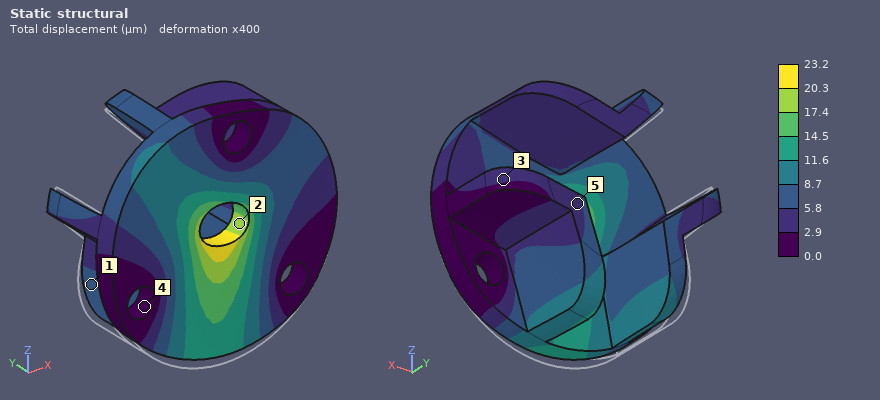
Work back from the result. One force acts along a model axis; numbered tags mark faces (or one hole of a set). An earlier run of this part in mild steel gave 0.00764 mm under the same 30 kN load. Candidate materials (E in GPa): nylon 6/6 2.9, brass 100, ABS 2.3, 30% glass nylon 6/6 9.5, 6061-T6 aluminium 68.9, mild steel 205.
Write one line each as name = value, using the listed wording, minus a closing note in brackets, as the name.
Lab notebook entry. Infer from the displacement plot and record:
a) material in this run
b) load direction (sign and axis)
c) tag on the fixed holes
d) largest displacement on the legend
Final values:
material in this run = 6061-T6 aluminium
load direction = +Z
tag on the fixed holes = 4
largest displacement on the legend = 23.2 µm
